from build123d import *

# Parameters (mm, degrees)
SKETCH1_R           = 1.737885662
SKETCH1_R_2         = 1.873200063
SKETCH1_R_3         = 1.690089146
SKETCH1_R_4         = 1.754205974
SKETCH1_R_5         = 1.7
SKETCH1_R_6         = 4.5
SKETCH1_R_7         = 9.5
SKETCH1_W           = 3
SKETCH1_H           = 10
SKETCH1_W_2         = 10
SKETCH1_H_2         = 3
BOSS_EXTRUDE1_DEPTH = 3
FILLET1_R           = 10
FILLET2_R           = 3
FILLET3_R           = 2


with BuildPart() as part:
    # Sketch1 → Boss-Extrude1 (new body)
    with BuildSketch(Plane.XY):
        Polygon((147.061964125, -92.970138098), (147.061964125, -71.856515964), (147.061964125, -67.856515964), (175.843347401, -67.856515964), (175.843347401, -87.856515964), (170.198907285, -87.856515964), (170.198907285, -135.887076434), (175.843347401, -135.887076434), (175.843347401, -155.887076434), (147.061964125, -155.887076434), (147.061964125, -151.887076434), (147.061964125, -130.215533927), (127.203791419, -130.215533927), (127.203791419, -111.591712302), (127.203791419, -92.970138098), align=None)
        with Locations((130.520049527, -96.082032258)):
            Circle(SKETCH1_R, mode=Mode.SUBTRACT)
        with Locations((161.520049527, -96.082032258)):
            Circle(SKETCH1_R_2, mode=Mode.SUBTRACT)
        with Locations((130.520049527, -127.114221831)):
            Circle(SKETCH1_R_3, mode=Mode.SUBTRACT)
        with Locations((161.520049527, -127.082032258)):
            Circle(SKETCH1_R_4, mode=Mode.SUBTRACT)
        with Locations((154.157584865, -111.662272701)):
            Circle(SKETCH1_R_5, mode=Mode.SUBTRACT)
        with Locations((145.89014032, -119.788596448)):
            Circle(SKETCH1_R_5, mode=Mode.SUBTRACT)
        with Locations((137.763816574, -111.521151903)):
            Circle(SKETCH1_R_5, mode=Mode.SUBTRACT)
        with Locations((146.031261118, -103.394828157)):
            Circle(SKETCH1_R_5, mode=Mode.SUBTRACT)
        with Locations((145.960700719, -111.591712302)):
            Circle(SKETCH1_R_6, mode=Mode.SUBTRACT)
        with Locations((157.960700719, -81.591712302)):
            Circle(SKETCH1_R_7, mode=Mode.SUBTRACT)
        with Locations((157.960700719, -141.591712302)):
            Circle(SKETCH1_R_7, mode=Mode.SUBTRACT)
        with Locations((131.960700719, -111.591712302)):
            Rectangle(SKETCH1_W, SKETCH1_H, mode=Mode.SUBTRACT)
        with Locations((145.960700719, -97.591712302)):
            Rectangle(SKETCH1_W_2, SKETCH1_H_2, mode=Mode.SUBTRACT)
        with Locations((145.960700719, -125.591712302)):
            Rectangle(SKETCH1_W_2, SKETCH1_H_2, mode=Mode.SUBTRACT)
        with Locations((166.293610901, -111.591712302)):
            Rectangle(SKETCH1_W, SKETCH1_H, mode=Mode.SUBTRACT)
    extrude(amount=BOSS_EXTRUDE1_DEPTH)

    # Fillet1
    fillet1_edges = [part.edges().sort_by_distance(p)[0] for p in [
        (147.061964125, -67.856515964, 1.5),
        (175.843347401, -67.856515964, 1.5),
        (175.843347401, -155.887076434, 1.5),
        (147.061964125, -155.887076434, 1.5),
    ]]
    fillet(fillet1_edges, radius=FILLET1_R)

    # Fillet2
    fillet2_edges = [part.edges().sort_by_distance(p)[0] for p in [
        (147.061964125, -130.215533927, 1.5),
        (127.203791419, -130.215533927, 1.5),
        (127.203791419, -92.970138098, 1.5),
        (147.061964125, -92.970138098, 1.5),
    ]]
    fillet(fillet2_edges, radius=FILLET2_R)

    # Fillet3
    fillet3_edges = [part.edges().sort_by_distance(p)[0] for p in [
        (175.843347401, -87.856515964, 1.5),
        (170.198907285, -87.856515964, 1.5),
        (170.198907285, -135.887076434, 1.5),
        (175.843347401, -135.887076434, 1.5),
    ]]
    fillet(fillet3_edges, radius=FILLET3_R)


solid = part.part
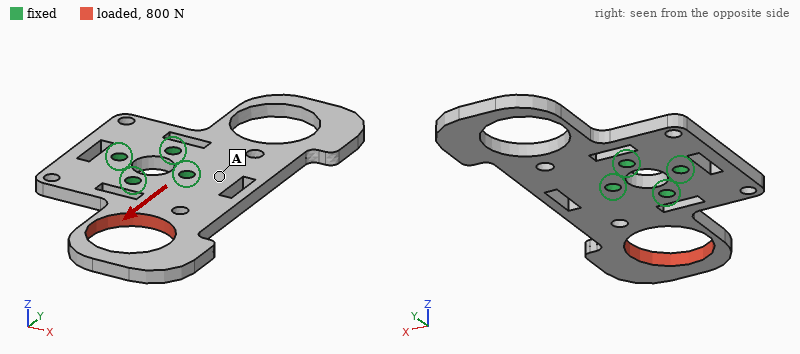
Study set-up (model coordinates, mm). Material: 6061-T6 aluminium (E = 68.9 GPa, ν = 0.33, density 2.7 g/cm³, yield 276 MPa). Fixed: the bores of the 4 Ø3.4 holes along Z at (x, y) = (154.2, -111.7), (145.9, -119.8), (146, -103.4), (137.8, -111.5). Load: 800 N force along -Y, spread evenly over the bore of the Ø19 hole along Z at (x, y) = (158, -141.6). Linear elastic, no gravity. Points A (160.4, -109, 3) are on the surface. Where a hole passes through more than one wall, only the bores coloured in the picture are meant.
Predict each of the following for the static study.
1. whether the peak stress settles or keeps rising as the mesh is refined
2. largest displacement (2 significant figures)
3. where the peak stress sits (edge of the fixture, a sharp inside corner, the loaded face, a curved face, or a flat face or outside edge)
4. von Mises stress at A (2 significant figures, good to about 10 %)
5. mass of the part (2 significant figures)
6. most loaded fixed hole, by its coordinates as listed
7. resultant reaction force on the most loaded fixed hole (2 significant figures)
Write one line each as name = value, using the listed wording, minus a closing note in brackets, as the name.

whether the peak stress settles or keeps rising as the mesh is refined = keeps rising
largest displacement = 27 µm
where the peak stress sits = a sharp inside corner
von Mises stress at A = 11 MPa
mass of the part = 17 g
most loaded fixed hole, by its coordinates as listed = (154.2, -111.7)
resultant reaction force on the most loaded fixed hole = 670 N
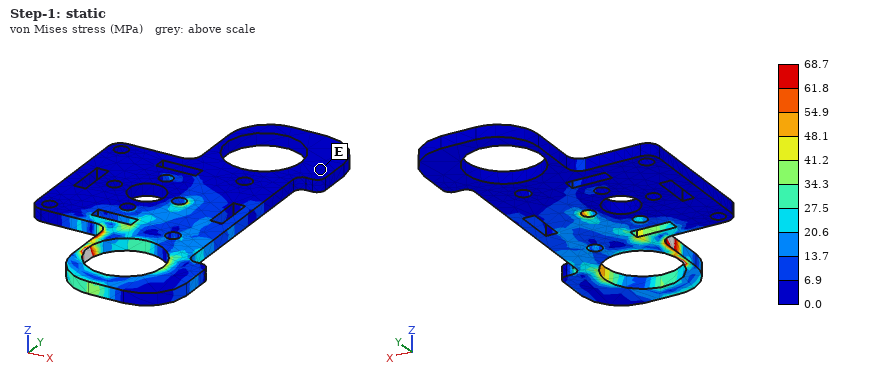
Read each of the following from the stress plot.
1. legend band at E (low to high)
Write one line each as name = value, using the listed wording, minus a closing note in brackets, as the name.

legend band at E = 0.0 to 6.9 MPa
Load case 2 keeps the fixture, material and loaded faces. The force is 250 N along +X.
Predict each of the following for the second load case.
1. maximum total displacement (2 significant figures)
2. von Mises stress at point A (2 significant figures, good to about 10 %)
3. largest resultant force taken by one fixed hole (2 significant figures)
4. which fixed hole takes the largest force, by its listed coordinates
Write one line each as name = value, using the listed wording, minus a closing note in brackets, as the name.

maximum total displacement = 61 µm
von Mises stress at point A = 7.2 MPa
largest resultant force taken by one fixed hole = 380 N
which fixed hole takes the largest force, by its listed coordinates = (145.9, -119.8)
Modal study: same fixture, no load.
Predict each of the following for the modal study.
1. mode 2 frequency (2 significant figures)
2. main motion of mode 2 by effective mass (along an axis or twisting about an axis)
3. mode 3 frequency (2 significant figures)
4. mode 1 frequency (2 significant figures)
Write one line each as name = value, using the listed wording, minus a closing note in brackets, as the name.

mode 2 frequency = 1500 Hz
main motion of mode 2 by effective mass = along Z
mode 3 frequency = 3900 Hz
mode 1 frequency = 1400 Hz
